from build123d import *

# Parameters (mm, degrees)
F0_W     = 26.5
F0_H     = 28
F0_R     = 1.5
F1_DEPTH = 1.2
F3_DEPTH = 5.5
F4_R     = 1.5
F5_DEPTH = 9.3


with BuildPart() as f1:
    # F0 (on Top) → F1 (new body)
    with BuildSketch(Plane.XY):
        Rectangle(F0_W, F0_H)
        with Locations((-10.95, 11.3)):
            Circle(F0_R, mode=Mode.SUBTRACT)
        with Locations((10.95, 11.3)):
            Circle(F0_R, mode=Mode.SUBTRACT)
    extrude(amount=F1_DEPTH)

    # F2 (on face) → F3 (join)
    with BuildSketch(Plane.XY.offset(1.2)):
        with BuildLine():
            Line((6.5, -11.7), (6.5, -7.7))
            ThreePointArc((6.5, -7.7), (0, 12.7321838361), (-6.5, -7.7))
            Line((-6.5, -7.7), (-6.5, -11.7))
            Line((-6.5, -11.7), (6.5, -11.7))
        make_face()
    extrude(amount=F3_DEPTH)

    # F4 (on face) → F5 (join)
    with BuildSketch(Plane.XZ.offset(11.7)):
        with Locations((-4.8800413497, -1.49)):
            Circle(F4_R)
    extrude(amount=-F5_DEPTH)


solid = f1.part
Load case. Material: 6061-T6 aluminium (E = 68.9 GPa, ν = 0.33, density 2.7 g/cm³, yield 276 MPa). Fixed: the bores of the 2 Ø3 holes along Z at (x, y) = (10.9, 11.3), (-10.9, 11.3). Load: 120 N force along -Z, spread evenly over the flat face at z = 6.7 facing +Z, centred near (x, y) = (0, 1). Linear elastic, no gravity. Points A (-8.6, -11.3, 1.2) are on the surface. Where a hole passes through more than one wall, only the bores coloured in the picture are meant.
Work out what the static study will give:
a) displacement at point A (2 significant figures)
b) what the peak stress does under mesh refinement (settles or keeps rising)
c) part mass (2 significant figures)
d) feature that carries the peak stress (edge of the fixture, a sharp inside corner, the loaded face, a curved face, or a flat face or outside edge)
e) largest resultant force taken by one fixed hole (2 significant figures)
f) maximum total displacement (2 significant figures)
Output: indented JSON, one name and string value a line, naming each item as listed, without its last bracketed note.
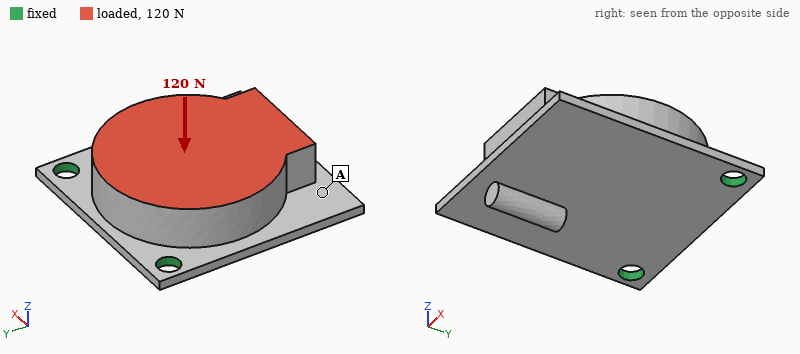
{
  "displacement at point A": "0.21 mm",
  "what the peak stress does under mesh refinement": "keeps rising",
  "part mass": "8.9 g",
  "feature that carries the peak stress": "edge of the fixture",
  "largest resultant force taken by one fixed hole": "62 N",
  "maximum total displacement": "0.23 mm"
}
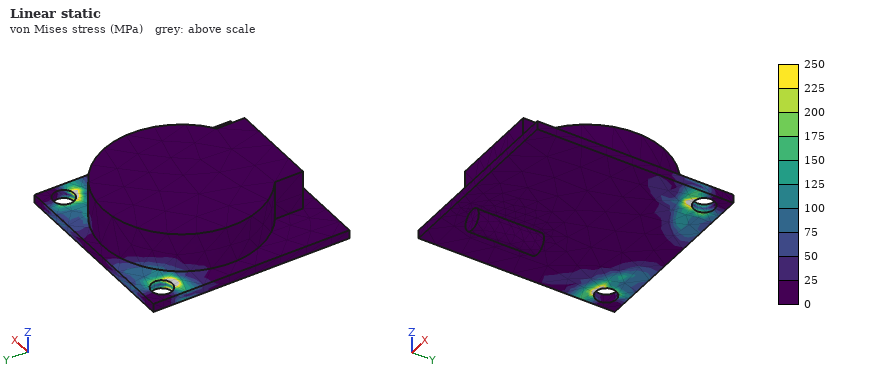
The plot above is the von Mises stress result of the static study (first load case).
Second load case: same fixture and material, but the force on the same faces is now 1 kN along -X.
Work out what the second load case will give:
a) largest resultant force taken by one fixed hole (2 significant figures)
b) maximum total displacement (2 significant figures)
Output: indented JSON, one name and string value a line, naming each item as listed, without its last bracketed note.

{
  "largest resultant force taken by one fixed hole": "760 N",
  "maximum total displacement": "30 µm"
}
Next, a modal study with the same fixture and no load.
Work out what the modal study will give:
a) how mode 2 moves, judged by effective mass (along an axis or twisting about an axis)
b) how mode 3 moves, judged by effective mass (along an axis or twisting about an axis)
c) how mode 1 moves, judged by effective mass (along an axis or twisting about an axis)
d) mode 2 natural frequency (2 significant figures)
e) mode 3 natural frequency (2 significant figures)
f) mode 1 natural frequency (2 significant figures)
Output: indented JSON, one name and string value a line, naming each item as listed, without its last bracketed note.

{
  "how mode 2 moves, judged by effective mass": "twisting about Y",
  "how mode 3 moves, judged by effective mass": "along X",
  "how mode 1 moves, judged by effective mass": "along Z",
  "mode 2 natural frequency": "13 kHz",
  "mode 3 natural frequency": "15 kHz",
  "mode 1 natural frequency": "1500 Hz"
}
